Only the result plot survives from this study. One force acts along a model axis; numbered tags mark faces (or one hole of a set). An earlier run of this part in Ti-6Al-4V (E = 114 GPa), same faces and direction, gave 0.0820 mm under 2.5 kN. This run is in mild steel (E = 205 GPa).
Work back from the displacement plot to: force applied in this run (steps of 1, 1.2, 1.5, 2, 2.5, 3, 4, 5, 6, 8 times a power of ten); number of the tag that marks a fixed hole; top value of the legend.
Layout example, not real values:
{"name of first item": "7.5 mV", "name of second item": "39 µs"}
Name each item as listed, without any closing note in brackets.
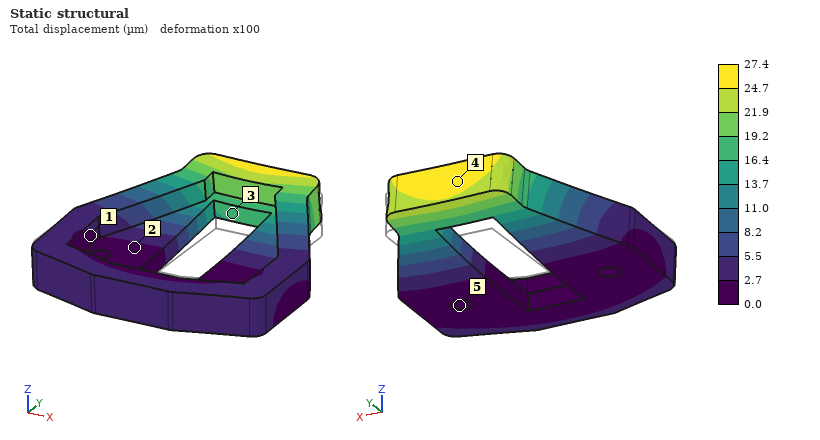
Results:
{"force applied in this run": "1.5 kN", "number of the tag that marks a fixed hole": "5", "top value of the legend": "27.4 µm"}
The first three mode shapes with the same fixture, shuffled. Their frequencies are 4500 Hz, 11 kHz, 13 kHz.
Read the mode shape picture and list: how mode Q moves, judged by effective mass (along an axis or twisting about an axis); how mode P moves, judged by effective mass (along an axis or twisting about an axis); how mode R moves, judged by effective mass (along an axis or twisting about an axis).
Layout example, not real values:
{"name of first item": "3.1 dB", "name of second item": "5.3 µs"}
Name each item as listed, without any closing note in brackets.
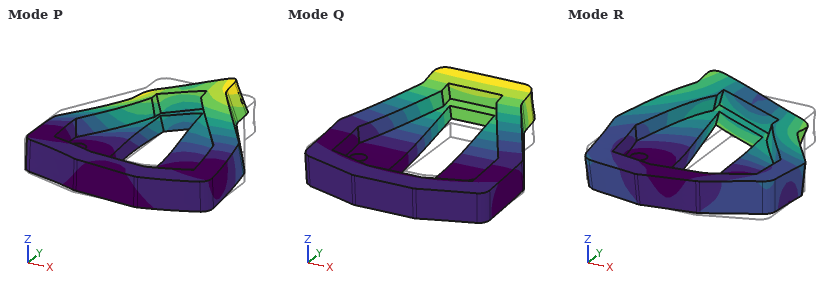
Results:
{"how mode Q moves, judged by effective mass": "along Z", "how mode P moves, judged by effective mass": "along X", "how mode R moves, judged by effective mass": "along X"}
